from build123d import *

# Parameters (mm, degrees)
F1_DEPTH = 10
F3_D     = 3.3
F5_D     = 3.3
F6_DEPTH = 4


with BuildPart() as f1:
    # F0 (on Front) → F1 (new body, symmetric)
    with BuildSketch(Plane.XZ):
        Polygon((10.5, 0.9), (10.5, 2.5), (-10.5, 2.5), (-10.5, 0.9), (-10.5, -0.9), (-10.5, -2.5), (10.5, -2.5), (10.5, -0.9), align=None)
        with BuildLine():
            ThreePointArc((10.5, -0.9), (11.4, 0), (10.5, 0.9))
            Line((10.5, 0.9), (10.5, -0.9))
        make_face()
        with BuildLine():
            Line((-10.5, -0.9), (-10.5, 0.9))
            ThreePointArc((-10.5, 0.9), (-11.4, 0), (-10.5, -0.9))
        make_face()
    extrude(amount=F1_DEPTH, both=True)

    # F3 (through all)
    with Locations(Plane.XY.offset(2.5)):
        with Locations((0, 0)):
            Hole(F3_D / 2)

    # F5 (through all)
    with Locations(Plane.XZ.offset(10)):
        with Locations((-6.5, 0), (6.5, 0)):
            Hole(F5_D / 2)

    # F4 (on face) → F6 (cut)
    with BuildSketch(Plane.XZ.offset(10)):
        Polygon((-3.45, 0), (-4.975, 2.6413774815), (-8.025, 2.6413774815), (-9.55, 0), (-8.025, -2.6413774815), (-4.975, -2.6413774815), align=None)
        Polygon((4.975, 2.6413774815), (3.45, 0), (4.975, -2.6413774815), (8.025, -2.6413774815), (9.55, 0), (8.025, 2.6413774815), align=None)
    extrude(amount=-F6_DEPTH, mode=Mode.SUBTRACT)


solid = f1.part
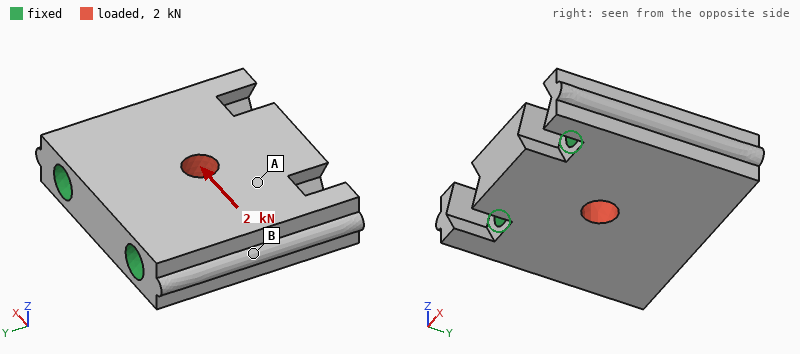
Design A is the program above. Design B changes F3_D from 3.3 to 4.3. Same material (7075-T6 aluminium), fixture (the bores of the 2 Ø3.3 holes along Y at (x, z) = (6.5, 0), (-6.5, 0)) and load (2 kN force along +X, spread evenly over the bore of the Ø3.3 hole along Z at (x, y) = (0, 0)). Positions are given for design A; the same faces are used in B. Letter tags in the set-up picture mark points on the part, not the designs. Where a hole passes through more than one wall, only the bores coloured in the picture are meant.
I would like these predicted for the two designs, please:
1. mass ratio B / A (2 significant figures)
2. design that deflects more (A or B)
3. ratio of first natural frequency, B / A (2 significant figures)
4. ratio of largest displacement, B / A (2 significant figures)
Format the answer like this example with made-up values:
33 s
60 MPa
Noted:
0.98
A
0.99
0.84
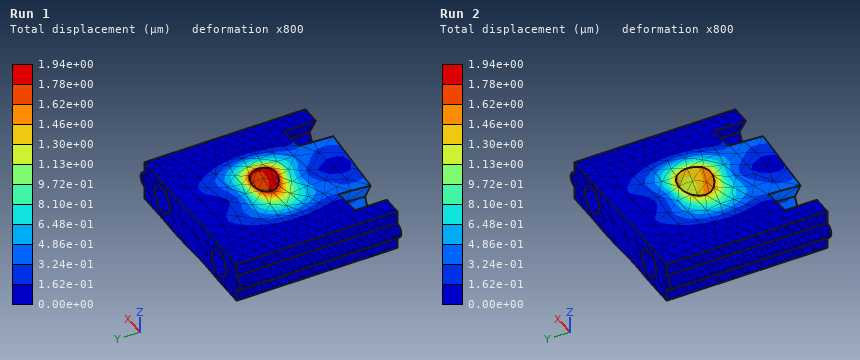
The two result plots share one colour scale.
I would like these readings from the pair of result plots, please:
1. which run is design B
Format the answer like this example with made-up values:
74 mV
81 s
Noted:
Run 2
